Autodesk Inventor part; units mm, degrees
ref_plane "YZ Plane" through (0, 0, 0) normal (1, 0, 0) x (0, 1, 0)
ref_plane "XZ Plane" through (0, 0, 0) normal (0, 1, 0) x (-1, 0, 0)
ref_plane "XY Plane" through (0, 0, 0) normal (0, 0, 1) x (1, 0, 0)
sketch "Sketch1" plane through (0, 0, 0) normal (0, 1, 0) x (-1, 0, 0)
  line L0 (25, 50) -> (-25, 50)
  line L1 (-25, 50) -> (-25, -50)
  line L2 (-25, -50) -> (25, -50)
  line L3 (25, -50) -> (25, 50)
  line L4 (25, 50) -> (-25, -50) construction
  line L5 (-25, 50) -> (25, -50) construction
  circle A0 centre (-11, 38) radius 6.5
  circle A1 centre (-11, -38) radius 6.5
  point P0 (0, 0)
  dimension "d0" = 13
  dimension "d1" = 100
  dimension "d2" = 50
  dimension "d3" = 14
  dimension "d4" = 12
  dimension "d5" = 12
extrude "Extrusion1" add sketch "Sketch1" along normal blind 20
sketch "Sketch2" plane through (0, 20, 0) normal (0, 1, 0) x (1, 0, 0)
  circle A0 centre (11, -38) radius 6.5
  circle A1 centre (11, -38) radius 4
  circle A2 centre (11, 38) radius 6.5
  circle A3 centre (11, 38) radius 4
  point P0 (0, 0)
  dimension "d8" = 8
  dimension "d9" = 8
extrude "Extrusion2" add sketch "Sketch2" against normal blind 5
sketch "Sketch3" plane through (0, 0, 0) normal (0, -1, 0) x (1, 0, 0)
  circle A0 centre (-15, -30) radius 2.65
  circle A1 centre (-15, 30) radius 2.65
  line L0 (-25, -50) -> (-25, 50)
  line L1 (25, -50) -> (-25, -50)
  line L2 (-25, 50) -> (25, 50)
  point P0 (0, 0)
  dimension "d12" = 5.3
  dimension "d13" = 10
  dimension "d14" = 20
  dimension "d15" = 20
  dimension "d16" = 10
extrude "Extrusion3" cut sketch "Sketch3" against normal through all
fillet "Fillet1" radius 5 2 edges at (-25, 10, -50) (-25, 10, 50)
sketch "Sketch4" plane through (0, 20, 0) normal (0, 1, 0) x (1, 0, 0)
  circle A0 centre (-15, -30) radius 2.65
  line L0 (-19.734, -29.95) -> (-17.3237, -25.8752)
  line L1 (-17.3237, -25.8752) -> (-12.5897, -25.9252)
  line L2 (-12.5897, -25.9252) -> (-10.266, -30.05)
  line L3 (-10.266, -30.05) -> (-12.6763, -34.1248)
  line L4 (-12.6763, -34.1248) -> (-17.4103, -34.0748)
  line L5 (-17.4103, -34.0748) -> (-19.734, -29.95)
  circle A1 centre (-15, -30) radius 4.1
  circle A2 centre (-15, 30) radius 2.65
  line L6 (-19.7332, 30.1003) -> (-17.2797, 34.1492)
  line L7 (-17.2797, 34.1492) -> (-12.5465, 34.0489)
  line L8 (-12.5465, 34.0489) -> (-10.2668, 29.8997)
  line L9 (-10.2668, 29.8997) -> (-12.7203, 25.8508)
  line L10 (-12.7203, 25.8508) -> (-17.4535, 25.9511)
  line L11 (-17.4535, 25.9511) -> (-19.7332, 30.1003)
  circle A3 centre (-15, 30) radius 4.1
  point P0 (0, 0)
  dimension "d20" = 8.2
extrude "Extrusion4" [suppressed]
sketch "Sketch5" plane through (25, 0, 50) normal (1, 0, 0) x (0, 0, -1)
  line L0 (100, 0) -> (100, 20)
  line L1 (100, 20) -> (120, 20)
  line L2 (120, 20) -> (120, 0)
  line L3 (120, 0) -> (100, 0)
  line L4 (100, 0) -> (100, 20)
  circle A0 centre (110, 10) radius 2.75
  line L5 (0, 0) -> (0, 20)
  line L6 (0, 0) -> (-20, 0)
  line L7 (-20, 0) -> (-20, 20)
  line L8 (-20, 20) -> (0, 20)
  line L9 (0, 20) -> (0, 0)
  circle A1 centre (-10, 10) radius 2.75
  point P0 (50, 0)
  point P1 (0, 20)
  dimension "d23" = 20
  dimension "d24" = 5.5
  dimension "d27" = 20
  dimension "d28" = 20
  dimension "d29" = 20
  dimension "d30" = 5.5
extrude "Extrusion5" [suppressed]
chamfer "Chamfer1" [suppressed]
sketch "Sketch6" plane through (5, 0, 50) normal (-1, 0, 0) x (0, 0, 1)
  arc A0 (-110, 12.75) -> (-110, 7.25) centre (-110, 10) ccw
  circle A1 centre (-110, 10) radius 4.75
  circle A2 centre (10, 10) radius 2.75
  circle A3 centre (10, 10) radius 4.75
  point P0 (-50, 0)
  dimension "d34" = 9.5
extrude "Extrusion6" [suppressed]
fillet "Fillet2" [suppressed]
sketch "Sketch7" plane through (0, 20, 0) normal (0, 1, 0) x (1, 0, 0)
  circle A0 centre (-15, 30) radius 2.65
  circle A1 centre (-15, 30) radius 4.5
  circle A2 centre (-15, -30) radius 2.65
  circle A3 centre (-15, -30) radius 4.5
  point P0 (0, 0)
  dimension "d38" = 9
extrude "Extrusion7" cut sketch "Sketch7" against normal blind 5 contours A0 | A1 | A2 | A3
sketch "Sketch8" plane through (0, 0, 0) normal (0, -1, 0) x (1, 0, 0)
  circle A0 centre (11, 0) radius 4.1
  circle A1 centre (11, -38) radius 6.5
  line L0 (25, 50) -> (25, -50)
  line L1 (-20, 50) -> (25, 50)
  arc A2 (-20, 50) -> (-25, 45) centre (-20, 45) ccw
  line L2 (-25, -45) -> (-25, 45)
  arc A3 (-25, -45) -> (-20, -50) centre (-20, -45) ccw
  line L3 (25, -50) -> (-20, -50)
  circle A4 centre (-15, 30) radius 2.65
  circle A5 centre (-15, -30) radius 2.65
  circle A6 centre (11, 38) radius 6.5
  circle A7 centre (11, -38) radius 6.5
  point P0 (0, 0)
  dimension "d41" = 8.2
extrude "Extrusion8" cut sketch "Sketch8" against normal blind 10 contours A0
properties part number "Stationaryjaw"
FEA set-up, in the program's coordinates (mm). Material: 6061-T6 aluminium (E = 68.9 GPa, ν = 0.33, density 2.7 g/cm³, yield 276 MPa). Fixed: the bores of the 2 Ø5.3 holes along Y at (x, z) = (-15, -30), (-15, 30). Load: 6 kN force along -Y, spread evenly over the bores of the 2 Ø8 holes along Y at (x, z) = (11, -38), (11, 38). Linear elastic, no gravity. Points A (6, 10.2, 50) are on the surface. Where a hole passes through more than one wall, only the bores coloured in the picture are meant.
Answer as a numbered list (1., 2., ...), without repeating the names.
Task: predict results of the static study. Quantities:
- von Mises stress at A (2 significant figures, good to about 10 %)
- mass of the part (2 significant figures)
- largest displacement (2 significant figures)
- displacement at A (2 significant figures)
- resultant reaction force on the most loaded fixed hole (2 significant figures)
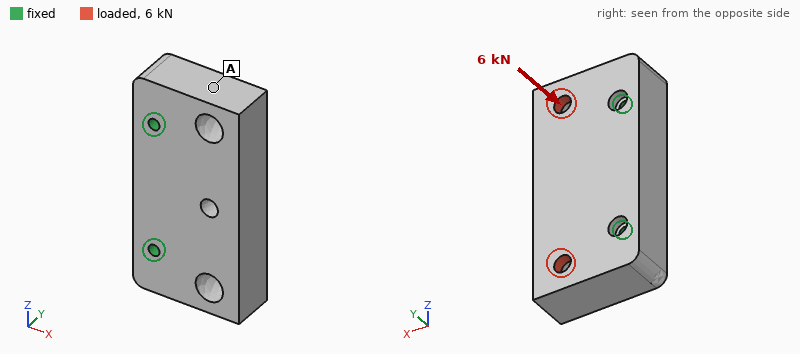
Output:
1. 15 MPa
2. 250 g
3. 63 µm
4. 33 µm
5. 3.0 kN
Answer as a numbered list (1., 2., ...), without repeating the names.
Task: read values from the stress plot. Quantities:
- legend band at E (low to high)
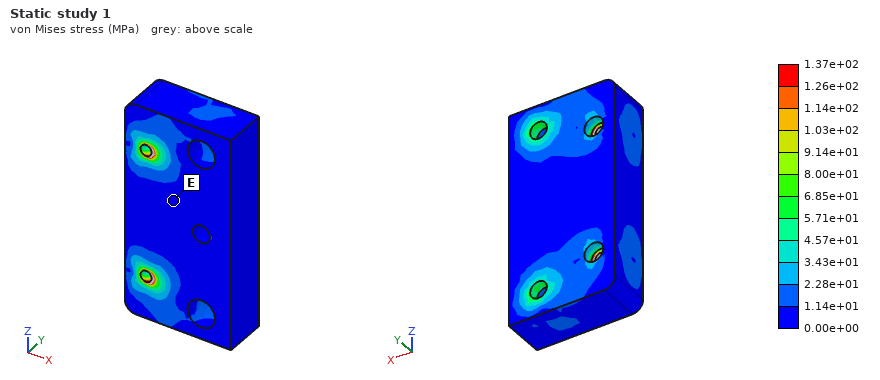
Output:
1. 0.00e+00 to 1.14e+01 MPa
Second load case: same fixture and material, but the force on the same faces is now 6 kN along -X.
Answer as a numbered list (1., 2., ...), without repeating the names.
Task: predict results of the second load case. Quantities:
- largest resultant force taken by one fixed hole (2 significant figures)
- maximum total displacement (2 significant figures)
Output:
1. 3.0 kN
2. 26 µm
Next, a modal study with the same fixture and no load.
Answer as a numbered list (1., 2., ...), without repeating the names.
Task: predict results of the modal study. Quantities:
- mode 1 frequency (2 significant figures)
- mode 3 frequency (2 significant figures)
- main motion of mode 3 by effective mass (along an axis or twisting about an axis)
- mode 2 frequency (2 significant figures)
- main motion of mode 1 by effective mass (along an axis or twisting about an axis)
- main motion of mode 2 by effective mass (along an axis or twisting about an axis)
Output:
1. 4900 Hz
2. 12 kHz
3. along Z
4. 8400 Hz
5. along Y
6. twisting about X
